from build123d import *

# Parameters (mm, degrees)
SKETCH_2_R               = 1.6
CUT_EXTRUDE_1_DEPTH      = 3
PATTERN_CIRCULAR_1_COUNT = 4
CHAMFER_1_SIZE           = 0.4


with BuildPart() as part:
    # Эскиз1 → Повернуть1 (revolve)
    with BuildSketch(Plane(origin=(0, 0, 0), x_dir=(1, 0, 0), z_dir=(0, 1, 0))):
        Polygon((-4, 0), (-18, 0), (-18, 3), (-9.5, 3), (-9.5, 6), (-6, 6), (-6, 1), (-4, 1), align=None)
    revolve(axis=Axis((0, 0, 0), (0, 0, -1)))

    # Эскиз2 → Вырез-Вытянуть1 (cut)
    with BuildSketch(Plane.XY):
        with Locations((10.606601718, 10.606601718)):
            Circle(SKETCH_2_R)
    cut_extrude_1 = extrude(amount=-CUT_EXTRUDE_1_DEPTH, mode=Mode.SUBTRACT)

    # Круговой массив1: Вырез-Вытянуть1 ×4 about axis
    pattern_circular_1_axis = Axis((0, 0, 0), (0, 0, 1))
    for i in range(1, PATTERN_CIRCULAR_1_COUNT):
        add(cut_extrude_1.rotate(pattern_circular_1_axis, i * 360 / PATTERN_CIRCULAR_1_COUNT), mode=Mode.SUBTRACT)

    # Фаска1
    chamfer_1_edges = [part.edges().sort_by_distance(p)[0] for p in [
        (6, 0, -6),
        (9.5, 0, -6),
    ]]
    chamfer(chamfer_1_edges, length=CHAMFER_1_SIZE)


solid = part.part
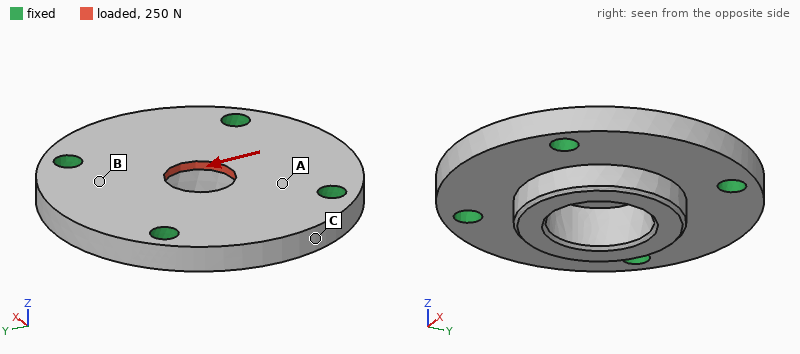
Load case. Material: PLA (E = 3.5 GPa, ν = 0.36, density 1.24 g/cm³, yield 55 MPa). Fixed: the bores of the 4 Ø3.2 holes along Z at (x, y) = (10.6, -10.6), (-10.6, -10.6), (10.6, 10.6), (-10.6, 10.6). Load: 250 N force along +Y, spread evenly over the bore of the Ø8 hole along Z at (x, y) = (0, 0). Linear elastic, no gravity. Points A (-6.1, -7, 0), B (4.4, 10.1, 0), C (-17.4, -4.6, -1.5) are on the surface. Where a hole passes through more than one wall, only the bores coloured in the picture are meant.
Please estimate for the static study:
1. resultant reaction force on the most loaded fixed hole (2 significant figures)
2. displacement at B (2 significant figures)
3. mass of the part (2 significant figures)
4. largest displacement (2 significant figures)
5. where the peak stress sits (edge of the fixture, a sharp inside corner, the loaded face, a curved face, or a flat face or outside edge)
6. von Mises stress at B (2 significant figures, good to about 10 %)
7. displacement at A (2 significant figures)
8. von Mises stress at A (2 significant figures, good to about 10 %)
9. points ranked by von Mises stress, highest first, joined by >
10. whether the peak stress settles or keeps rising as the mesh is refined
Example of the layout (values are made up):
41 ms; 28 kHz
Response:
66 N; 7.5 µm; 3.9 g; 24 µm; a sharp inside corner; 2.7 MPa; 6.0 µm; 4.3 MPa; A > B > C; keeps rising
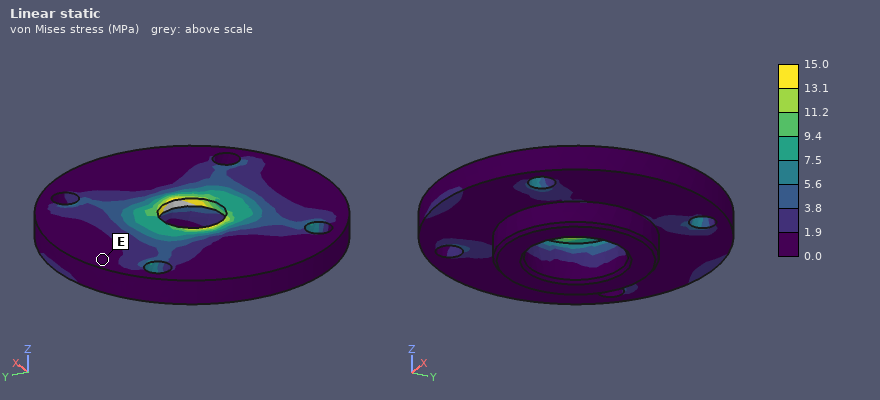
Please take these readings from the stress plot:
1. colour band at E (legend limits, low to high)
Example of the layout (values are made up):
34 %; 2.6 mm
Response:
0.0 to 1.9 MPa
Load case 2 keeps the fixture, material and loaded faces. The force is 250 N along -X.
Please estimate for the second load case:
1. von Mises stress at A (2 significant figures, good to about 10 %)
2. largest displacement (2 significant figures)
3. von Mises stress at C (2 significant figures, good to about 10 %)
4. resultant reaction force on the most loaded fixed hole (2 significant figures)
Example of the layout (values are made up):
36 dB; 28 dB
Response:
3.9 MPa; 24 µm; 1.6 MPa; 66 N
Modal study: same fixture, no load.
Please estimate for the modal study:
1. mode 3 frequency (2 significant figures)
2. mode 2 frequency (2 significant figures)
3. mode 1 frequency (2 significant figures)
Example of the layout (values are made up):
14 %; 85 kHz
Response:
10 kHz; 9800 Hz; 9700 Hz
